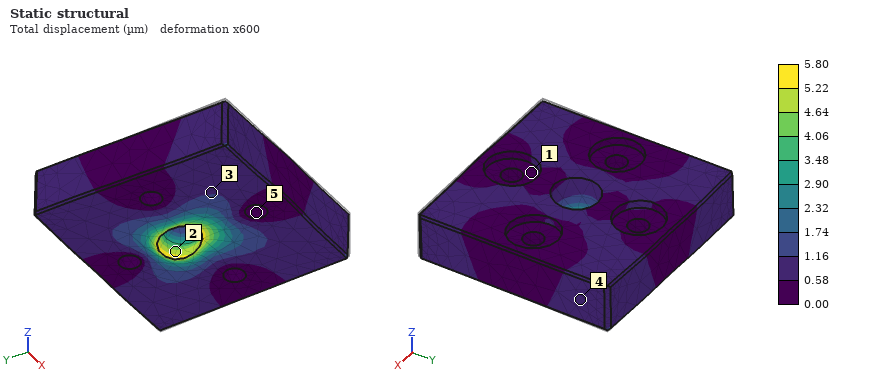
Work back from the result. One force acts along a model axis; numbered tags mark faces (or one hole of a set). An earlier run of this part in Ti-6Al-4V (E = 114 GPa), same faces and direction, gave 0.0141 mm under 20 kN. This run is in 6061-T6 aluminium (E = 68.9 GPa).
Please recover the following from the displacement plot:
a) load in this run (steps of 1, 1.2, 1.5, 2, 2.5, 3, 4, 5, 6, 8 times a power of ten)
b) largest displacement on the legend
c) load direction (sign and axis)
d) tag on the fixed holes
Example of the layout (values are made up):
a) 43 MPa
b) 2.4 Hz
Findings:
a) 5 kN
b) 5.80 µm
c) +Y
d) 5
